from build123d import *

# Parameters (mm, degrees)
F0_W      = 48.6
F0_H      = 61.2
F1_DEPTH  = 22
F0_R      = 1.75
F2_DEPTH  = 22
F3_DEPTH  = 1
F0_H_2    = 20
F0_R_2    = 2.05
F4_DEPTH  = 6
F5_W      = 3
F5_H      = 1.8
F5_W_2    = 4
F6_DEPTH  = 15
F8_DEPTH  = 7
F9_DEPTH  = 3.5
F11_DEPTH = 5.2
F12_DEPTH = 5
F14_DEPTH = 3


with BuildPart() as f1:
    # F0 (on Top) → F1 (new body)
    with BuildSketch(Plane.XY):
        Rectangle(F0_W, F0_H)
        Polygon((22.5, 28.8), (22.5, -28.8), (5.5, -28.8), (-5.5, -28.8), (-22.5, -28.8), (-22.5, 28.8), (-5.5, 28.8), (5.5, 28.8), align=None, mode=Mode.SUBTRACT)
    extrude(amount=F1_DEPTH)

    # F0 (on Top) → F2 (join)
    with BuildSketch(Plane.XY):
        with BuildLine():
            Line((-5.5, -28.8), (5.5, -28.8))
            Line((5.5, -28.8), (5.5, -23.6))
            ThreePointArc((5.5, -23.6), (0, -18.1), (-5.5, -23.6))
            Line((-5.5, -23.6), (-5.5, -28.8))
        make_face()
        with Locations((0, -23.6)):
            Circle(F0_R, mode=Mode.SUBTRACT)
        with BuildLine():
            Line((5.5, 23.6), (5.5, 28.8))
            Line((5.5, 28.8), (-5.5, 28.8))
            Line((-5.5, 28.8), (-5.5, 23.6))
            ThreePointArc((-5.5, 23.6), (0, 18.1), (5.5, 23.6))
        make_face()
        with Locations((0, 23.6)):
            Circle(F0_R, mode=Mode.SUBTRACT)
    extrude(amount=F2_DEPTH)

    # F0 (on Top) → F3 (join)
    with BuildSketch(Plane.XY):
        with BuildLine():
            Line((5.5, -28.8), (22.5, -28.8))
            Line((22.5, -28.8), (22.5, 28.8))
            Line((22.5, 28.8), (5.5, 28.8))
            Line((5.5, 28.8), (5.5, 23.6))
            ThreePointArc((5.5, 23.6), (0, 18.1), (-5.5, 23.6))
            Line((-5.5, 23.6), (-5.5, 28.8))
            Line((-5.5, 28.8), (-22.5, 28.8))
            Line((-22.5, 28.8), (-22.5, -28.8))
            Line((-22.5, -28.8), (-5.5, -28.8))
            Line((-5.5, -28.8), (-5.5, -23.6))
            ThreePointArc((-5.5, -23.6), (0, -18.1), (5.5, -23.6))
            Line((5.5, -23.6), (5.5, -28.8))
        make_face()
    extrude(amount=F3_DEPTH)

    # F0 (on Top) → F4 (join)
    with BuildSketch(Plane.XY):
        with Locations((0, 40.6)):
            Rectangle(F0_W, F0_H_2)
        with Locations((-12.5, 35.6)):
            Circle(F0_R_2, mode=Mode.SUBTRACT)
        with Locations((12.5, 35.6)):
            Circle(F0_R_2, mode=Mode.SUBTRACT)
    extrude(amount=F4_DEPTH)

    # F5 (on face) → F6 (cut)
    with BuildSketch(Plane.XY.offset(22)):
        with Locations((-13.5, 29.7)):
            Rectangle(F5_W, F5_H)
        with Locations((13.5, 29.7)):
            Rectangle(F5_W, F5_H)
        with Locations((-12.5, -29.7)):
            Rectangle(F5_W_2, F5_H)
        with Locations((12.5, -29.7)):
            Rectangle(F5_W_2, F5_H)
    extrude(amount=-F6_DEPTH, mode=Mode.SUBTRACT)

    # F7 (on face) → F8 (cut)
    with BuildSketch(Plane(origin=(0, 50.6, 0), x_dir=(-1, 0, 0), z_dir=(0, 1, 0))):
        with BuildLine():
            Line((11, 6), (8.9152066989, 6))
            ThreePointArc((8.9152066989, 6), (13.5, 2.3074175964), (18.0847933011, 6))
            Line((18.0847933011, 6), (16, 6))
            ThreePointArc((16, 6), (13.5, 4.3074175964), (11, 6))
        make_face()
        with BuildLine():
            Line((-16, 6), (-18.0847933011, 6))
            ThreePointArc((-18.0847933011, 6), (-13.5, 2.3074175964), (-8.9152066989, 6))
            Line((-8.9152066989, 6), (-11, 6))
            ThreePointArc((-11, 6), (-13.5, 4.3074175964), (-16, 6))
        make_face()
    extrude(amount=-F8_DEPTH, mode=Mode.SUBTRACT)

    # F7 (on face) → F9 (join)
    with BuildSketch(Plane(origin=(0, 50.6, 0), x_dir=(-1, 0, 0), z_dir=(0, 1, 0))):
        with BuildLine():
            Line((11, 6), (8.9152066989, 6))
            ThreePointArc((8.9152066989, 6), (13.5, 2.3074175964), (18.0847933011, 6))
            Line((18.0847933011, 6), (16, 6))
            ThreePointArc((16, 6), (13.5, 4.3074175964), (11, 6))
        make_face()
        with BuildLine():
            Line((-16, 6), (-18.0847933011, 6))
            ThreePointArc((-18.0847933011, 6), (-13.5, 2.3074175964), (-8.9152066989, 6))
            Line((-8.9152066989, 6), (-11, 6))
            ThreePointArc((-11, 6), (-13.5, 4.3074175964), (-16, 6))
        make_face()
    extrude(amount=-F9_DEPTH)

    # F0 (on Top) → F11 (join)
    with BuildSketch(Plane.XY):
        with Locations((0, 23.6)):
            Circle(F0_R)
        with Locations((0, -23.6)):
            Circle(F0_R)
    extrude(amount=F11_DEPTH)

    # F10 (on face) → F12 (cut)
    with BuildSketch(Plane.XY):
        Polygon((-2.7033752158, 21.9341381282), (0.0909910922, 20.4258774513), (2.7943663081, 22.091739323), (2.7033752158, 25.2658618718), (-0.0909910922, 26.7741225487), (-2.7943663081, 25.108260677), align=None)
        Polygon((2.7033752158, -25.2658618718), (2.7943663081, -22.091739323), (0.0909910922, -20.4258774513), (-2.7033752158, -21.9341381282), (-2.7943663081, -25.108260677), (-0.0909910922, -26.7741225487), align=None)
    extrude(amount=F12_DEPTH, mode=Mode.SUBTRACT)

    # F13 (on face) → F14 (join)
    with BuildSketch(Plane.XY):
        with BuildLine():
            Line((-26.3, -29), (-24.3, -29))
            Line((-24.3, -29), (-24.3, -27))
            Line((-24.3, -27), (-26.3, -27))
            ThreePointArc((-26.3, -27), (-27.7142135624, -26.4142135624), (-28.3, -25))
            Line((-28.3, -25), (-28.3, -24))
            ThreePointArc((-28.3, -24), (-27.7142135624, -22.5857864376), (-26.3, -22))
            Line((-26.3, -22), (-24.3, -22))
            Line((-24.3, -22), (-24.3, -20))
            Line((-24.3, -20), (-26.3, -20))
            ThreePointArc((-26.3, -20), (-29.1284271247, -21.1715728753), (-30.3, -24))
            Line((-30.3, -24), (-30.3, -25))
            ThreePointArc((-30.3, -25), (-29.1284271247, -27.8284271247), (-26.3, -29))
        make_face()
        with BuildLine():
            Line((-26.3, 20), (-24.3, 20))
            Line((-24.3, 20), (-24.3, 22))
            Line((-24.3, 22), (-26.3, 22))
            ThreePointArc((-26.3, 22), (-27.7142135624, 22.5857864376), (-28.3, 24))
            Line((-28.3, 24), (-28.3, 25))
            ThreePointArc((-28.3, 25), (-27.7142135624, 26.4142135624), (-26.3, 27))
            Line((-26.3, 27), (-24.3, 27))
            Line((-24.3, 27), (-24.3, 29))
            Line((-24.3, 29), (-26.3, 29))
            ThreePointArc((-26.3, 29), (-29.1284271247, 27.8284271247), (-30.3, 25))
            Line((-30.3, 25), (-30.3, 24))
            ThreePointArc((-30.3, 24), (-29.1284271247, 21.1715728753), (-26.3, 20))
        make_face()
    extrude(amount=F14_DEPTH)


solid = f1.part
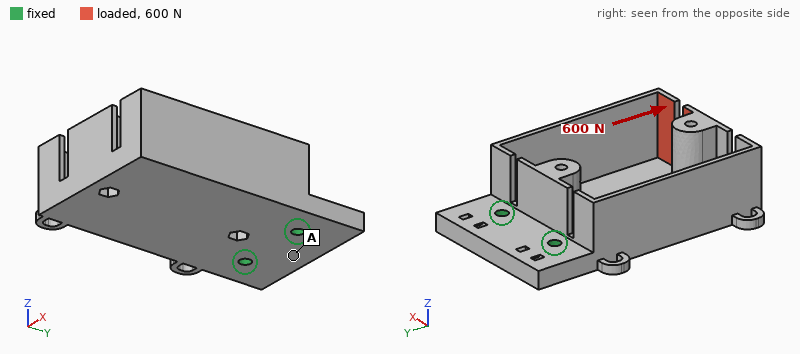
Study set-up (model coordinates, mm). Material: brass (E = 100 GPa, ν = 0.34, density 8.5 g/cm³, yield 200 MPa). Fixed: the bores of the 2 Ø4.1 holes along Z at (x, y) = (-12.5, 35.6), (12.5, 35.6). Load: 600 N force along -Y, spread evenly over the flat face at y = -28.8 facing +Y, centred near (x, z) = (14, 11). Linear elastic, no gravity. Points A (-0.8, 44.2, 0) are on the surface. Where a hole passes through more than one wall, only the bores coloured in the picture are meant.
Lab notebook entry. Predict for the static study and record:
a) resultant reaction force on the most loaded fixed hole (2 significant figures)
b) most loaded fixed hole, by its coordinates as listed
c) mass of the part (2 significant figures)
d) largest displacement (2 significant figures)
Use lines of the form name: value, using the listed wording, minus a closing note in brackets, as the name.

resultant reaction force on the most loaded fixed hole: 600 N
most loaded fixed hole, by its coordinates as listed: (12.5, 35.6)
mass of the part: 170 g
largest displacement: 0.36 mm
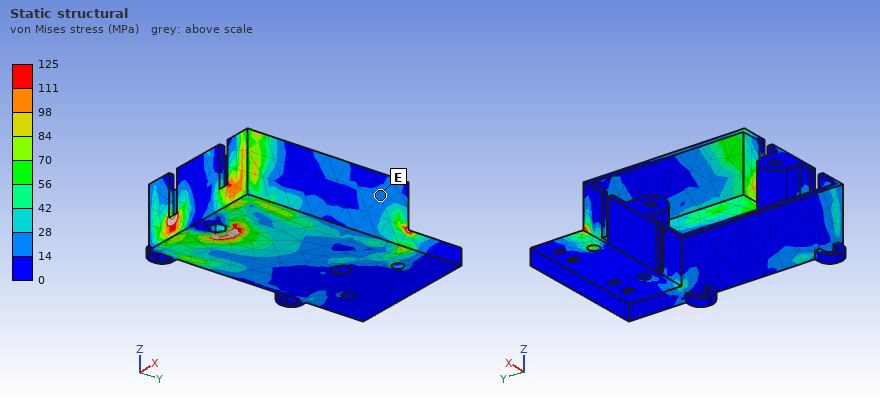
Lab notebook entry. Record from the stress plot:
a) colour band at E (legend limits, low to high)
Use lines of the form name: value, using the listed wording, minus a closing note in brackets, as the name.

colour band at E: 14 to 28 MPa
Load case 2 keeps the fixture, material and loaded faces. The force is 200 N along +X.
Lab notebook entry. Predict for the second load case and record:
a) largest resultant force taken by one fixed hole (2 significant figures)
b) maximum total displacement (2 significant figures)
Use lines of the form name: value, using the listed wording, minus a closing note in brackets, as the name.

largest resultant force taken by one fixed hole: 490 N
maximum total displacement: 0.24 mm
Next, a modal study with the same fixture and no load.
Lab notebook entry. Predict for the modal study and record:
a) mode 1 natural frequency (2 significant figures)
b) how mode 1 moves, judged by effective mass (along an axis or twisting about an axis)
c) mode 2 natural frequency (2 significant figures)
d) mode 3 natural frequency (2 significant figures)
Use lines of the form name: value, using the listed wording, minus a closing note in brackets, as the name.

mode 1 natural frequency: 540 Hz
how mode 1 moves, judged by effective mass: along Z
mode 2 natural frequency: 670 Hz
mode 3 natural frequency: 1200 Hz
